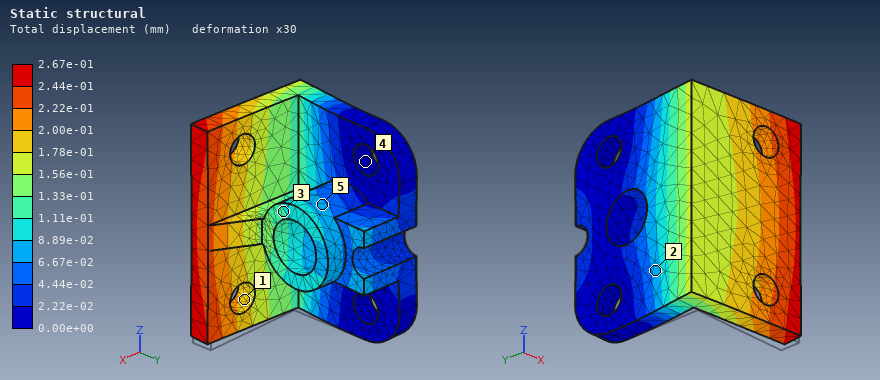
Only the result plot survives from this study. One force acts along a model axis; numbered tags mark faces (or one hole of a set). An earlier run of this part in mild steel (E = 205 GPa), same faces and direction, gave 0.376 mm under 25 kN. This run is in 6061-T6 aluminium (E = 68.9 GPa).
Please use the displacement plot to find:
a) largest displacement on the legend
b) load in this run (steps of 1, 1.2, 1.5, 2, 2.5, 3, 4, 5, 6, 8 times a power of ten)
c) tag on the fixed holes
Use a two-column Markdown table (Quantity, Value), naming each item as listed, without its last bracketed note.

| Quantity | Value |
|---|---|
| largest displacement on the legend | 2.67e-01 mm |
| load in this run | 6 kN |
| tag on the fixed holes | 4 |
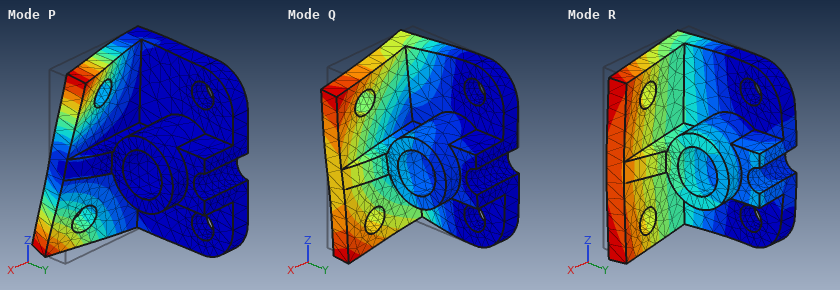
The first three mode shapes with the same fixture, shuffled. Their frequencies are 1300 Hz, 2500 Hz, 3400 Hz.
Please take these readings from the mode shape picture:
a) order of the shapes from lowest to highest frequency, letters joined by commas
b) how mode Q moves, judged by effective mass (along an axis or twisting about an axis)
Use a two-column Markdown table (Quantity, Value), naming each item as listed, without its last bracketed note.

| Quantity | Value |
|---|---|
| order of the shapes from lowest to highest frequency, letters joined by commas | R, Q, P |
| how mode Q moves, judged by effective mass | along Z |
